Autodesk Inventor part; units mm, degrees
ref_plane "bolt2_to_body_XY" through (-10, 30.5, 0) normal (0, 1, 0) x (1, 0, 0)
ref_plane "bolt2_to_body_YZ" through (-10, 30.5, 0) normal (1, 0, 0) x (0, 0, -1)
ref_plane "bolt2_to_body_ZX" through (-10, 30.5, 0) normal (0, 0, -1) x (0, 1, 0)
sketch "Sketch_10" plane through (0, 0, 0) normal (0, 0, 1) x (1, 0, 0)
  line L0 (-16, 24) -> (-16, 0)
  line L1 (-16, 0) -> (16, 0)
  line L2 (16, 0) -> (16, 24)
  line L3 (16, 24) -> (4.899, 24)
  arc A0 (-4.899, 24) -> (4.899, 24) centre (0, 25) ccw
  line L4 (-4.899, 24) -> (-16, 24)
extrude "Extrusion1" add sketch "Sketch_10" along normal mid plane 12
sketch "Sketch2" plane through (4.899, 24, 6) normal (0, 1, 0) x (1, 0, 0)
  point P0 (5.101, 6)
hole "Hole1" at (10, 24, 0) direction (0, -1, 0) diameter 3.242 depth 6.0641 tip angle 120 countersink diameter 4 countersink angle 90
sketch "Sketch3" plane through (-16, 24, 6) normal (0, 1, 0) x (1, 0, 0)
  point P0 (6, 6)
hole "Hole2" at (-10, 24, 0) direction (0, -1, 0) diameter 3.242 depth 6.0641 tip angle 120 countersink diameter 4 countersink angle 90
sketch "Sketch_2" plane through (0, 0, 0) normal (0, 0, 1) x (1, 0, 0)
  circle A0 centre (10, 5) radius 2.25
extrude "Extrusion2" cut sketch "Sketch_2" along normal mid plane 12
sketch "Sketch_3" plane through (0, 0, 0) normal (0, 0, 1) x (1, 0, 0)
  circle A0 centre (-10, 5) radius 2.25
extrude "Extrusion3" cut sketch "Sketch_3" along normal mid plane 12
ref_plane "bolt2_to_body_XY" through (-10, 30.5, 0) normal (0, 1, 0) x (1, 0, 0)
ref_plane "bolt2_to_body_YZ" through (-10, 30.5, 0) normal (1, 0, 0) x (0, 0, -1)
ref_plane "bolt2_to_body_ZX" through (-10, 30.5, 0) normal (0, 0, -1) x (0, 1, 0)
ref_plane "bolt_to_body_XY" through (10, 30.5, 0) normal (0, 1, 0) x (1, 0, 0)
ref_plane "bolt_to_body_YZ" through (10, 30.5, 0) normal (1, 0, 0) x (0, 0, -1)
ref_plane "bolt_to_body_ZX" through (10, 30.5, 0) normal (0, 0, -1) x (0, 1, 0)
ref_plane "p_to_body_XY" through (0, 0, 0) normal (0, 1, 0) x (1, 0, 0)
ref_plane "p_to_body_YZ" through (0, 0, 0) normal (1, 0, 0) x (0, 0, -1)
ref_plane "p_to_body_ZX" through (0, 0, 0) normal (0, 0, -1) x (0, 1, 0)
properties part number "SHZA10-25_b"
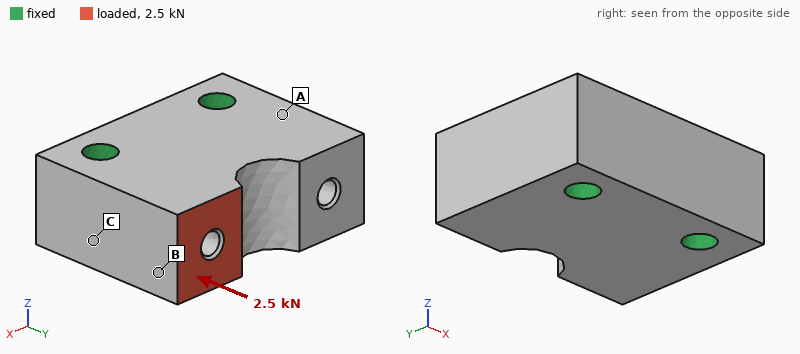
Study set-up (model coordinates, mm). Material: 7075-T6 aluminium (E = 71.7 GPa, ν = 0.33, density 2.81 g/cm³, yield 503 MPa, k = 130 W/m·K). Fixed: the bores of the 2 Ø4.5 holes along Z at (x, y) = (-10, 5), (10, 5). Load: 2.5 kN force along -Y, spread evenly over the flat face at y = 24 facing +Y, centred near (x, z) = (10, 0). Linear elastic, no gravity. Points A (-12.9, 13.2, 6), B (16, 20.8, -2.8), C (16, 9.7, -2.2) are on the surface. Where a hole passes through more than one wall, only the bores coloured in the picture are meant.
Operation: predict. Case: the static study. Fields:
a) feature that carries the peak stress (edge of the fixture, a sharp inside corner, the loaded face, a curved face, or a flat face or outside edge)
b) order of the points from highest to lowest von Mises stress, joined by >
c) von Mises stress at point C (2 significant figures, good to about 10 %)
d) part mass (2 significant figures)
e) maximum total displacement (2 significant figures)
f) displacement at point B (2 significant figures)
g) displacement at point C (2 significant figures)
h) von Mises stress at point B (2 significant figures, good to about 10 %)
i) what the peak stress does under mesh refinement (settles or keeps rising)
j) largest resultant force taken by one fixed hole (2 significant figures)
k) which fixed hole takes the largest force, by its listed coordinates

edge of the fixture
B > C > A
15 MPa
24 g
7.2 µm
5.9 µm
2.2 µm
22 MPa
keeps rising
2.4 kN
(10, 5)
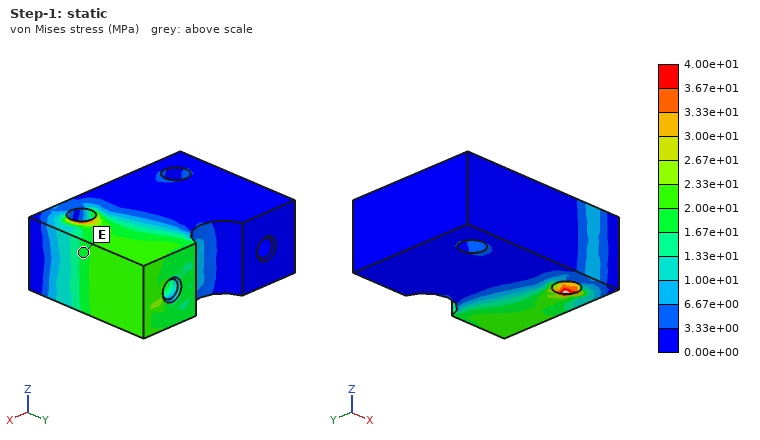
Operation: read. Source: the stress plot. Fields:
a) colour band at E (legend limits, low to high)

1.67e+01 to 2.00e+01 MPa
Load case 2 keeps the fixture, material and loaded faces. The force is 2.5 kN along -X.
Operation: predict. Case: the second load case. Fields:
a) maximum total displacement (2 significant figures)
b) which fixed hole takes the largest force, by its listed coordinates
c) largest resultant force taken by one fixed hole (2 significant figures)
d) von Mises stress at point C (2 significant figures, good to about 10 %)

22 µm
(-10, 5)
2.6 kN
28 MPa
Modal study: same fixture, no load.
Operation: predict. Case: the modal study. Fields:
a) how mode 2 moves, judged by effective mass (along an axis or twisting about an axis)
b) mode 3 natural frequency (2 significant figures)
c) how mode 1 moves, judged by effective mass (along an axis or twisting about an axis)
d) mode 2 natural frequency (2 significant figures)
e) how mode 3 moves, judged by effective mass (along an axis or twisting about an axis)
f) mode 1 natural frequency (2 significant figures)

twisting about Y
34 kHz
along Z
31 kHz
along X
22 kHz
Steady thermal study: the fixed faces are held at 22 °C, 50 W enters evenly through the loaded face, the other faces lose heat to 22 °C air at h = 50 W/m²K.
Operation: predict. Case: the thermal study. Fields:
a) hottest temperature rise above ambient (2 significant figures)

41 K
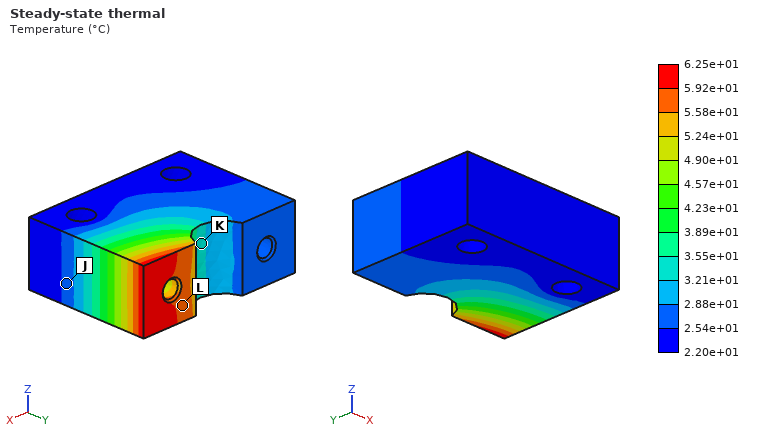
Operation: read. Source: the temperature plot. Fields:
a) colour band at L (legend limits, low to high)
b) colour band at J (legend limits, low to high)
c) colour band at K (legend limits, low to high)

5.58e+01 to 5.92e+01 °C
2.54e+01 to 2.88e+01 °C
3.21e+01 to 3.55e+01 °C
